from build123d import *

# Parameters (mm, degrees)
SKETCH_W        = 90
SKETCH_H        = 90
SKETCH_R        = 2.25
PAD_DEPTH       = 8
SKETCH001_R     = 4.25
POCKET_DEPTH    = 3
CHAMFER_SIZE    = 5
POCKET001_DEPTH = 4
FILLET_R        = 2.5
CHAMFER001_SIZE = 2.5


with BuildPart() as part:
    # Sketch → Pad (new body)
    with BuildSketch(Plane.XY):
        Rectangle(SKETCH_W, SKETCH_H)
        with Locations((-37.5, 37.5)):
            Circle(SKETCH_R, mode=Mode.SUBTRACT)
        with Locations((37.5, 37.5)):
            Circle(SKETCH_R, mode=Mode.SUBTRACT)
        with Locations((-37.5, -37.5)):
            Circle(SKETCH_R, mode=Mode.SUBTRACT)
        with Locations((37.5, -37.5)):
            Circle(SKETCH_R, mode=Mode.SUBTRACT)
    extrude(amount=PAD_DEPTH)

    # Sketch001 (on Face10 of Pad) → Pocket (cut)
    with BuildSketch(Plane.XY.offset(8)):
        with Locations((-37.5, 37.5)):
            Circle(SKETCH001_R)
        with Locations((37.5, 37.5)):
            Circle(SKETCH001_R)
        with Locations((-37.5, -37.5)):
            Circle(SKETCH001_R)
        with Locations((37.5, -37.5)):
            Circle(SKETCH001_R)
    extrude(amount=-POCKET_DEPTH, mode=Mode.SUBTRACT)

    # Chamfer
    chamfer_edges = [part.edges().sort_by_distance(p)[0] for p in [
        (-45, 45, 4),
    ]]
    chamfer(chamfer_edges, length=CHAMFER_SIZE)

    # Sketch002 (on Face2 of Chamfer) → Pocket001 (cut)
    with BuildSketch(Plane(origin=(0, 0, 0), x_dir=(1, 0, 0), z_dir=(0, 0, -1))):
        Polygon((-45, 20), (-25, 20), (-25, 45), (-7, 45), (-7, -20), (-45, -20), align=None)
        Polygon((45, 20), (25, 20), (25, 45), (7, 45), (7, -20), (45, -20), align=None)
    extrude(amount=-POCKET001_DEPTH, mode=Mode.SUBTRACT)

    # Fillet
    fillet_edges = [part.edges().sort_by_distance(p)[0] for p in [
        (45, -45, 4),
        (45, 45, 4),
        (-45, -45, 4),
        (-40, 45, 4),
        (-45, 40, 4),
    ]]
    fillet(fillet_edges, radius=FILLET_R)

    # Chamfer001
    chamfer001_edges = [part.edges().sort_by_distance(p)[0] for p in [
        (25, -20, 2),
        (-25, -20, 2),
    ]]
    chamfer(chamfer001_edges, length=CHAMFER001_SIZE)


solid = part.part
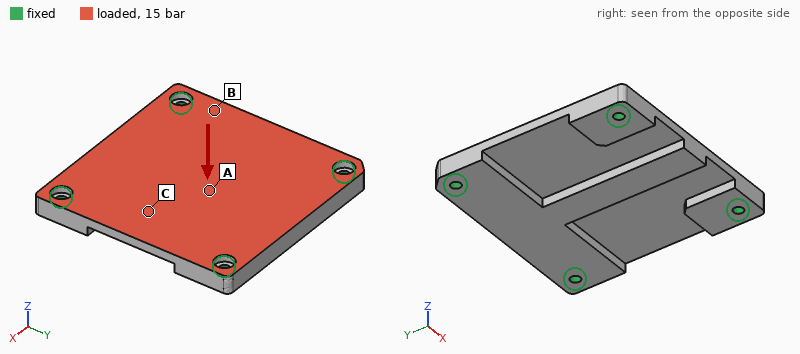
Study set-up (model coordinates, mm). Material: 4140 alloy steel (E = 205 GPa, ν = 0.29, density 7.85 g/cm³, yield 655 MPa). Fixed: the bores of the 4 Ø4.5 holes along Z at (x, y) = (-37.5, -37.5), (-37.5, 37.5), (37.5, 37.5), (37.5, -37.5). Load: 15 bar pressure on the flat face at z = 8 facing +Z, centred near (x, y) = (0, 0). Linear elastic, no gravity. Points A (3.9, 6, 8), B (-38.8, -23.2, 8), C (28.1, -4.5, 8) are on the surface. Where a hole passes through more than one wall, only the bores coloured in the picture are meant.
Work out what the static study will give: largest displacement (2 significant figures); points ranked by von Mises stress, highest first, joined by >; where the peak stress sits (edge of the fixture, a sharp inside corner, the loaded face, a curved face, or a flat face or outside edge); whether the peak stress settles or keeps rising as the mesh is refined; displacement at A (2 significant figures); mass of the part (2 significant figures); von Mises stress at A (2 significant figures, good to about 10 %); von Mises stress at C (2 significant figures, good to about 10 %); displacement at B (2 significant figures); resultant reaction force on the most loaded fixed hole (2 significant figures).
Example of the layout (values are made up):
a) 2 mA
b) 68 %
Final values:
a) 91 µm
b) C > A > B
c) edge of the fixture
d) keeps rising
e) 86 µm
f) 380 g
g) 64 MPa
h) 91 MPa
i) 19 µm
j) 5.7 kN
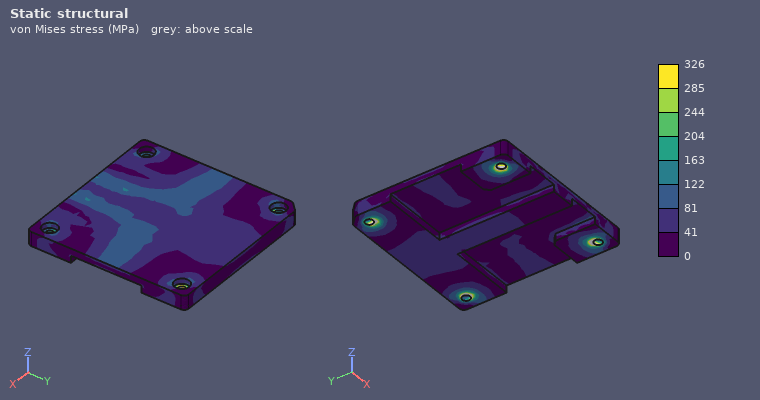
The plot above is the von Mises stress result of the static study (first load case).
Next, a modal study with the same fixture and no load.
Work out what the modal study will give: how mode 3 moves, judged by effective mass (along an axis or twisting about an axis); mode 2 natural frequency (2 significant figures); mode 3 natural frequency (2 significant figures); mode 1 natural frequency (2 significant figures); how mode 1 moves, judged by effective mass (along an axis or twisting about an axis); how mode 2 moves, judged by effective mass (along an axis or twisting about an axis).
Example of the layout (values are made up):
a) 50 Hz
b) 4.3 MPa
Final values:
a) twisting about Y
b) 5500 Hz
c) 6600 Hz
d) 3700 Hz
e) along Z
f) twisting about X
